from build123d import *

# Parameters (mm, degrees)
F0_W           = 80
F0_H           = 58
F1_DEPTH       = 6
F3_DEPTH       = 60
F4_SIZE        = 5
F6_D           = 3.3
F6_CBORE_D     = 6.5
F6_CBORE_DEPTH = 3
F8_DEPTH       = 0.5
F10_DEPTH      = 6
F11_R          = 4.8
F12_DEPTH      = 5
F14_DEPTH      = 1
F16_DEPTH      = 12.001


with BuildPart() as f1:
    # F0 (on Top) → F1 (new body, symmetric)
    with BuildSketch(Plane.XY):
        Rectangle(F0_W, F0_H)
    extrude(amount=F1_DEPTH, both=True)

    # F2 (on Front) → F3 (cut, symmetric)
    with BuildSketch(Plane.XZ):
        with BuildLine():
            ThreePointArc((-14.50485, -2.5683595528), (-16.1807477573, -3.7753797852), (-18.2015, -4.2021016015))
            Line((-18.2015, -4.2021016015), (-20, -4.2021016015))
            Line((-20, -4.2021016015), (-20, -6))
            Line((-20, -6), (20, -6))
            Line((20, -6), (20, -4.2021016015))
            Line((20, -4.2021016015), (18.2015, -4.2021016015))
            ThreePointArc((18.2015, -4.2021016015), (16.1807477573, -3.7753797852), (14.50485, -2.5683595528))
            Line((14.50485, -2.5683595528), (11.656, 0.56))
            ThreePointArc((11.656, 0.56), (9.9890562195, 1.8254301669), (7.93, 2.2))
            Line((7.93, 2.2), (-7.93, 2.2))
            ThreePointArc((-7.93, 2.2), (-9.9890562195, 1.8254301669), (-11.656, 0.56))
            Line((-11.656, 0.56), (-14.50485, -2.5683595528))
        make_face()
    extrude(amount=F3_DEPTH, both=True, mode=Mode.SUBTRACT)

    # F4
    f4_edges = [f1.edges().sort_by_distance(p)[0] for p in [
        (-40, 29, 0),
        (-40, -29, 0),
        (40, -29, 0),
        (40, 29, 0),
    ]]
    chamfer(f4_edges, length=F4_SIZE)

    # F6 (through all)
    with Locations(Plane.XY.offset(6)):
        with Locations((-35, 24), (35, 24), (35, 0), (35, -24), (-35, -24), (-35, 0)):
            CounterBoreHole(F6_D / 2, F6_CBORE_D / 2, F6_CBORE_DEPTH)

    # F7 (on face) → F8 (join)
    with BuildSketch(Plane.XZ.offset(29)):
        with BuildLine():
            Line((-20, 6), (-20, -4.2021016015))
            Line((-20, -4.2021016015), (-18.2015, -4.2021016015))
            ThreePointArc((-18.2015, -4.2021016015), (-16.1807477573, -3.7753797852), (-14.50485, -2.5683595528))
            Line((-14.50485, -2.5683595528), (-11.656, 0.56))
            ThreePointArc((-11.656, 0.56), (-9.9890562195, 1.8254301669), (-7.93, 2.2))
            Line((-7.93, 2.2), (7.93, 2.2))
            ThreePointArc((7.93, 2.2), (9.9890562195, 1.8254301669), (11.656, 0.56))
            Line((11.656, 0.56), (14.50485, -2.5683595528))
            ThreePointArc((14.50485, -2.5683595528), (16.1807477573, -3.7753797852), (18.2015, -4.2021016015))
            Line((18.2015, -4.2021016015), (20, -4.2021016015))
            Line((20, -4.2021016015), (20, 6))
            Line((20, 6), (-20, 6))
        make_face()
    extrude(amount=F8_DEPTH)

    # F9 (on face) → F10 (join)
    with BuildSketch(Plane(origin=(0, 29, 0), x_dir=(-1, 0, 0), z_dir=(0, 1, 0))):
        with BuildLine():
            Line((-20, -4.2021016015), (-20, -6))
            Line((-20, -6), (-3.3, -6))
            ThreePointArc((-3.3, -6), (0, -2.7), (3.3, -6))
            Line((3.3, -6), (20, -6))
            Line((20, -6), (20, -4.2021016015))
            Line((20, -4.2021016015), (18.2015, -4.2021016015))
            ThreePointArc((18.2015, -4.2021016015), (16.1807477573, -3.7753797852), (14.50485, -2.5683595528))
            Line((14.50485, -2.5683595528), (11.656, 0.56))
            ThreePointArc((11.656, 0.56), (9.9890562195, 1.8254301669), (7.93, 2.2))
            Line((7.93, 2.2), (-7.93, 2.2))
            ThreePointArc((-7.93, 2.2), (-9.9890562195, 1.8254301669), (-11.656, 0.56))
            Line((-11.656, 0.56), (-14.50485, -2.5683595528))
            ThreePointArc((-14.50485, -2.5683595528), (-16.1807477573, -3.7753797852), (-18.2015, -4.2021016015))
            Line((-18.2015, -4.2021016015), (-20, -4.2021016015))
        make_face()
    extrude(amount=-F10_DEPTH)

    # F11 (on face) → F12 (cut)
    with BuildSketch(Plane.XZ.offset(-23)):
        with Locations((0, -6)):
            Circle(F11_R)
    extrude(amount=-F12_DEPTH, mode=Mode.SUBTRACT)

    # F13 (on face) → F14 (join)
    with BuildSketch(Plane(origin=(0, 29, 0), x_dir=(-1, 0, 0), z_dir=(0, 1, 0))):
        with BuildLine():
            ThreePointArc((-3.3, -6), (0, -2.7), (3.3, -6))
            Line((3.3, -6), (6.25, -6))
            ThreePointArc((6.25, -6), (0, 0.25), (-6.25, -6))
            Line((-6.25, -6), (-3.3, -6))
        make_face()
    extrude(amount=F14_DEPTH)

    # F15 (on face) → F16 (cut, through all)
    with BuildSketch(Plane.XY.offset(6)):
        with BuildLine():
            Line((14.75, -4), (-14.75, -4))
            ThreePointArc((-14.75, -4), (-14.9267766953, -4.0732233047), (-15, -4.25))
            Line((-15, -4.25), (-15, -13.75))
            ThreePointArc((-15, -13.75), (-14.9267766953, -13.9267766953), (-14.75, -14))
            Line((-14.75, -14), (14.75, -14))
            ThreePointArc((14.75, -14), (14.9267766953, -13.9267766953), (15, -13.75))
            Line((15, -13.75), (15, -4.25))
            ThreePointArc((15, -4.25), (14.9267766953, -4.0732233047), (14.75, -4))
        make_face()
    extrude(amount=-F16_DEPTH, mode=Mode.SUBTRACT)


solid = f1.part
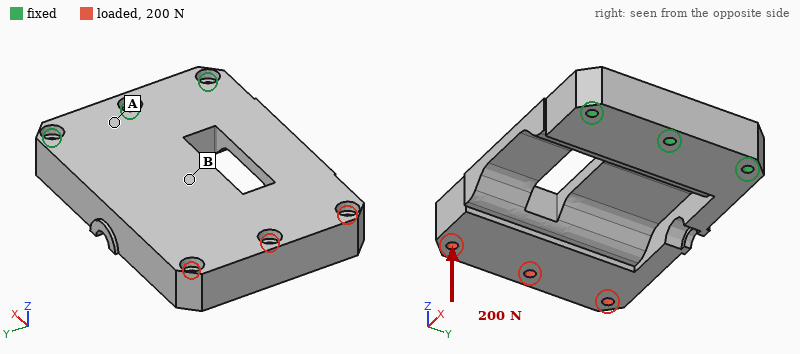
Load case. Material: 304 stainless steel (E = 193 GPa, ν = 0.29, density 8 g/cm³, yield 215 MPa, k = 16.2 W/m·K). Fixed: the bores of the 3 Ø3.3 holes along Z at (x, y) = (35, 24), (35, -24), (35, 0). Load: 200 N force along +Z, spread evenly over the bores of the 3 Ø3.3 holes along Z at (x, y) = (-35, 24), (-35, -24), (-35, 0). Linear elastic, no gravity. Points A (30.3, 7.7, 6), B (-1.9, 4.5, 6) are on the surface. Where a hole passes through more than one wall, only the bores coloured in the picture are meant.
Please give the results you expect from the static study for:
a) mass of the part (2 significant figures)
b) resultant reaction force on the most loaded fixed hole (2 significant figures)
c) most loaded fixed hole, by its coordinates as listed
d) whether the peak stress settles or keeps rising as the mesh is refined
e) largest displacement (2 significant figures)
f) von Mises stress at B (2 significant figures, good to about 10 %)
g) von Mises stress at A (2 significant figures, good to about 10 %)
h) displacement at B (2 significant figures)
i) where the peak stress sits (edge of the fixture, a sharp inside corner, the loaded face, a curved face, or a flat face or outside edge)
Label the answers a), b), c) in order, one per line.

a) 320 g
b) 240 N
c) (35, 0)
d) keeps rising
e) 87 µm
f) 21 MPa
g) 8.5 MPa
h) 18 µm
i) a sharp inside corner
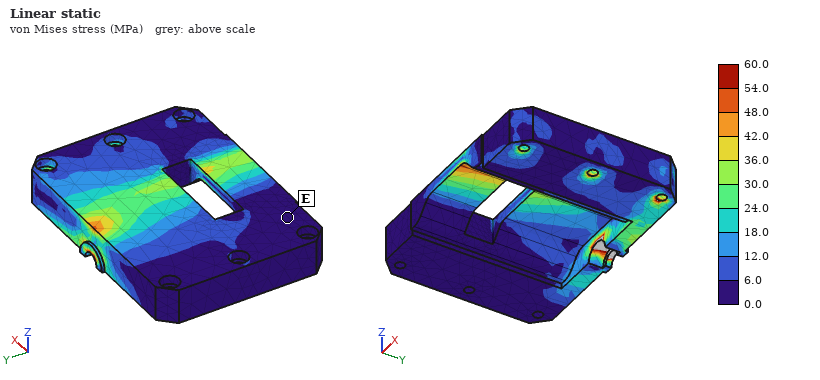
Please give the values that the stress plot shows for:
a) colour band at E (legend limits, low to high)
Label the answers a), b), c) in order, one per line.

a) 0.0 to 6.0 MPa
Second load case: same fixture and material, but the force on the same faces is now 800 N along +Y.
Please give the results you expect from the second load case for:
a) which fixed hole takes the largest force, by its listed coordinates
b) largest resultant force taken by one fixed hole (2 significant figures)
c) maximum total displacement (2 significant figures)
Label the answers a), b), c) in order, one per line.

a) (35, 24)
b) 1.3 kN
c) 26 µm
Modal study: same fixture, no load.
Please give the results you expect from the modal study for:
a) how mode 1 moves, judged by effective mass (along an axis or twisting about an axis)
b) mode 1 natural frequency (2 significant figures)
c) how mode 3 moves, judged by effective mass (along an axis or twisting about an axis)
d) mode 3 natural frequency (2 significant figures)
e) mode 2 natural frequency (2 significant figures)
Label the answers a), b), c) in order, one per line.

a) along Z
b) 850 Hz
c) along Y
d) 4400 Hz
e) 2500 Hz
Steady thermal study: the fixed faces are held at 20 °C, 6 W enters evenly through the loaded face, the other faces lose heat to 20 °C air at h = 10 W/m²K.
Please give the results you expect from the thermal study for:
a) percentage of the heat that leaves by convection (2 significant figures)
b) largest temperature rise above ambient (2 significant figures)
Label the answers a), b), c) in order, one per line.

a) 48 %
b) 51 K
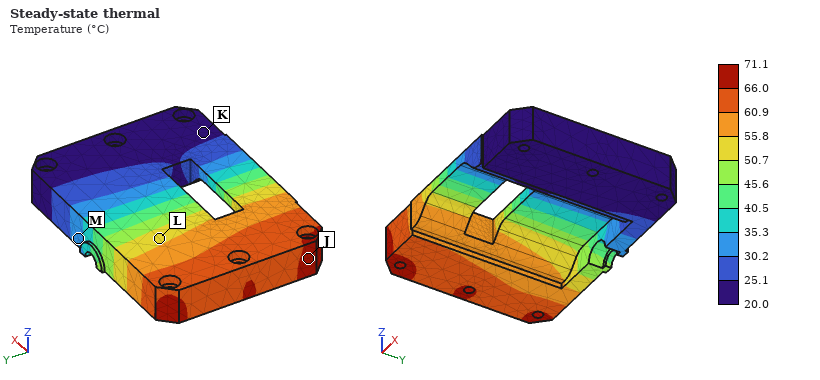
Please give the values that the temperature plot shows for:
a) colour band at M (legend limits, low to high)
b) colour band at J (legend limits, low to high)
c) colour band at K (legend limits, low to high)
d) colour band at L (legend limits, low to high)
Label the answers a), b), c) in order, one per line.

a) 30.2 to 35.3 °C
b) 66.0 to 71.1 °C
c) 20.0 to 25.1 °C
d) 50.7 to 55.8 °C
